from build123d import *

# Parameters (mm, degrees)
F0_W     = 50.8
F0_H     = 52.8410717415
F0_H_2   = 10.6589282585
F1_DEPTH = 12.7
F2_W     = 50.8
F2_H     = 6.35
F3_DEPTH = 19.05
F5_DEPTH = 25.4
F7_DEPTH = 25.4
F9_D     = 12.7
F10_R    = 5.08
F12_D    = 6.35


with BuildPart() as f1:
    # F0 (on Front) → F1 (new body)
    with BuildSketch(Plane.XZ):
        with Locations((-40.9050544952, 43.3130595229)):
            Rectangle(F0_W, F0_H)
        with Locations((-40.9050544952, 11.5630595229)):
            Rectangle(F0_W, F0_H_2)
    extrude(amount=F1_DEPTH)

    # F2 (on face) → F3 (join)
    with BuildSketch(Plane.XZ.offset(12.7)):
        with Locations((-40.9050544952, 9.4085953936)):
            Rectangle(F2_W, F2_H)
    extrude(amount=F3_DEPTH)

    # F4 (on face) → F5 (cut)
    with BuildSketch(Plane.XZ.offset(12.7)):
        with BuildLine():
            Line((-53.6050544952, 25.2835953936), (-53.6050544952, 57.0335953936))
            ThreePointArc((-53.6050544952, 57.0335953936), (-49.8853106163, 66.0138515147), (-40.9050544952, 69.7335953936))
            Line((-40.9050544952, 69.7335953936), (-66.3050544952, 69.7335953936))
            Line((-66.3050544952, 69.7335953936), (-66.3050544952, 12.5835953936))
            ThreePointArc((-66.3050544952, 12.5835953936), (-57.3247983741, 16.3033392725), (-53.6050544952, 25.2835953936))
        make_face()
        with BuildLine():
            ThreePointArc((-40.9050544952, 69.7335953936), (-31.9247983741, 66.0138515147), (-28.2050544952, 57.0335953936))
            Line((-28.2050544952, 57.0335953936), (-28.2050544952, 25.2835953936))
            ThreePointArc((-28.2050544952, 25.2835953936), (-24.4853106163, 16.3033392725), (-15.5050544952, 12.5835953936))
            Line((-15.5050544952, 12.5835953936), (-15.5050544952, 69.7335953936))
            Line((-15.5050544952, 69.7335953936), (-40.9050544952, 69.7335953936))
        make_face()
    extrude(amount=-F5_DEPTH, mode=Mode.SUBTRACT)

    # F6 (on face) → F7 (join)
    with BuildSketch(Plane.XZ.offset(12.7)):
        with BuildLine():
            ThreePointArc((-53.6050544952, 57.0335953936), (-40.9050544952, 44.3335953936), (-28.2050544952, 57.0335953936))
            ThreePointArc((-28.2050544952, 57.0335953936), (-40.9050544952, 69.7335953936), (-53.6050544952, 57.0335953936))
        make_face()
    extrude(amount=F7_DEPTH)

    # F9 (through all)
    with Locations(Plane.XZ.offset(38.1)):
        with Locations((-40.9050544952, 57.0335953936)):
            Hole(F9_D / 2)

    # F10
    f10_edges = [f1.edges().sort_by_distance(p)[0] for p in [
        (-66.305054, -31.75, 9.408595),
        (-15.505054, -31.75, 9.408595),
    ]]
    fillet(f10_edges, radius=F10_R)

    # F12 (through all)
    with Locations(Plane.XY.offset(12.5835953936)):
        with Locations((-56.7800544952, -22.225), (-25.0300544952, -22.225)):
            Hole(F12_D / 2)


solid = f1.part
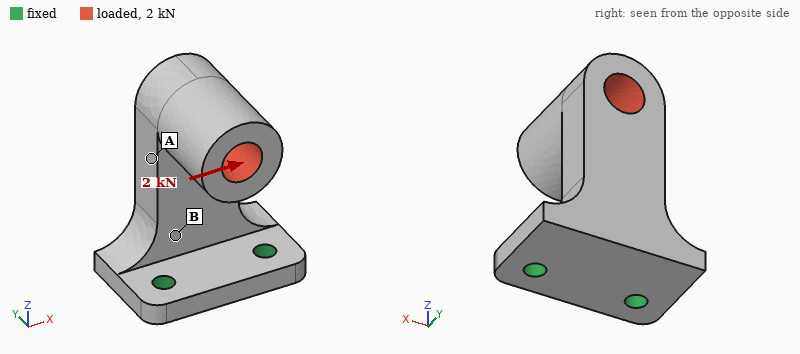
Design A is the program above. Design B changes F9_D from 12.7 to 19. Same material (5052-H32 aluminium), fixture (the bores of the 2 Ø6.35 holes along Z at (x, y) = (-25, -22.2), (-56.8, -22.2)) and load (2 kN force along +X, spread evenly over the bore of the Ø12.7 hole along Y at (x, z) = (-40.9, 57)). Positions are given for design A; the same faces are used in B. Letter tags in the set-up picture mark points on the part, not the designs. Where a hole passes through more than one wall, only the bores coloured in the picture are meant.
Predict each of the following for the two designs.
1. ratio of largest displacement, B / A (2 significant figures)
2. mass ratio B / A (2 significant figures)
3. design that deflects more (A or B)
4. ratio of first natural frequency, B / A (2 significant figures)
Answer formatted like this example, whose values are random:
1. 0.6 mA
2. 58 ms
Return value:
1. 1.1
2. 0.84
3. B
4. 1.2
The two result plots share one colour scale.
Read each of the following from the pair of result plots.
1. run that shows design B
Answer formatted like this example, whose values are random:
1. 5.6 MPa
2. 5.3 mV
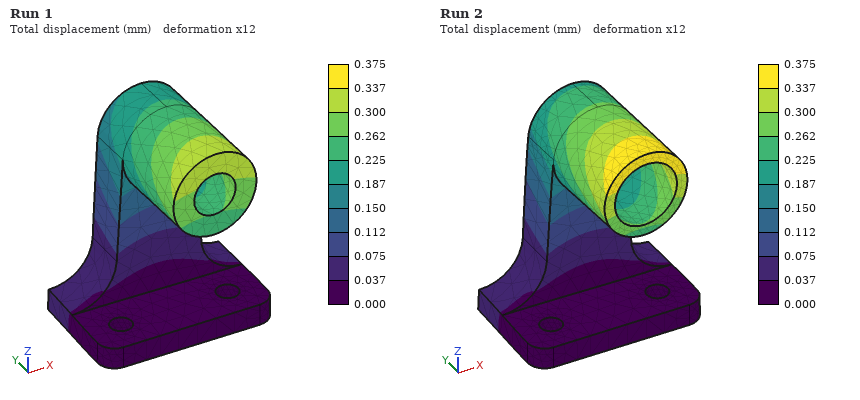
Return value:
1. Run 2
